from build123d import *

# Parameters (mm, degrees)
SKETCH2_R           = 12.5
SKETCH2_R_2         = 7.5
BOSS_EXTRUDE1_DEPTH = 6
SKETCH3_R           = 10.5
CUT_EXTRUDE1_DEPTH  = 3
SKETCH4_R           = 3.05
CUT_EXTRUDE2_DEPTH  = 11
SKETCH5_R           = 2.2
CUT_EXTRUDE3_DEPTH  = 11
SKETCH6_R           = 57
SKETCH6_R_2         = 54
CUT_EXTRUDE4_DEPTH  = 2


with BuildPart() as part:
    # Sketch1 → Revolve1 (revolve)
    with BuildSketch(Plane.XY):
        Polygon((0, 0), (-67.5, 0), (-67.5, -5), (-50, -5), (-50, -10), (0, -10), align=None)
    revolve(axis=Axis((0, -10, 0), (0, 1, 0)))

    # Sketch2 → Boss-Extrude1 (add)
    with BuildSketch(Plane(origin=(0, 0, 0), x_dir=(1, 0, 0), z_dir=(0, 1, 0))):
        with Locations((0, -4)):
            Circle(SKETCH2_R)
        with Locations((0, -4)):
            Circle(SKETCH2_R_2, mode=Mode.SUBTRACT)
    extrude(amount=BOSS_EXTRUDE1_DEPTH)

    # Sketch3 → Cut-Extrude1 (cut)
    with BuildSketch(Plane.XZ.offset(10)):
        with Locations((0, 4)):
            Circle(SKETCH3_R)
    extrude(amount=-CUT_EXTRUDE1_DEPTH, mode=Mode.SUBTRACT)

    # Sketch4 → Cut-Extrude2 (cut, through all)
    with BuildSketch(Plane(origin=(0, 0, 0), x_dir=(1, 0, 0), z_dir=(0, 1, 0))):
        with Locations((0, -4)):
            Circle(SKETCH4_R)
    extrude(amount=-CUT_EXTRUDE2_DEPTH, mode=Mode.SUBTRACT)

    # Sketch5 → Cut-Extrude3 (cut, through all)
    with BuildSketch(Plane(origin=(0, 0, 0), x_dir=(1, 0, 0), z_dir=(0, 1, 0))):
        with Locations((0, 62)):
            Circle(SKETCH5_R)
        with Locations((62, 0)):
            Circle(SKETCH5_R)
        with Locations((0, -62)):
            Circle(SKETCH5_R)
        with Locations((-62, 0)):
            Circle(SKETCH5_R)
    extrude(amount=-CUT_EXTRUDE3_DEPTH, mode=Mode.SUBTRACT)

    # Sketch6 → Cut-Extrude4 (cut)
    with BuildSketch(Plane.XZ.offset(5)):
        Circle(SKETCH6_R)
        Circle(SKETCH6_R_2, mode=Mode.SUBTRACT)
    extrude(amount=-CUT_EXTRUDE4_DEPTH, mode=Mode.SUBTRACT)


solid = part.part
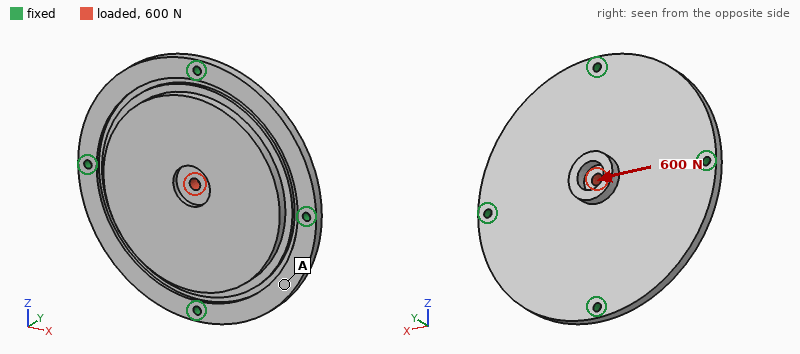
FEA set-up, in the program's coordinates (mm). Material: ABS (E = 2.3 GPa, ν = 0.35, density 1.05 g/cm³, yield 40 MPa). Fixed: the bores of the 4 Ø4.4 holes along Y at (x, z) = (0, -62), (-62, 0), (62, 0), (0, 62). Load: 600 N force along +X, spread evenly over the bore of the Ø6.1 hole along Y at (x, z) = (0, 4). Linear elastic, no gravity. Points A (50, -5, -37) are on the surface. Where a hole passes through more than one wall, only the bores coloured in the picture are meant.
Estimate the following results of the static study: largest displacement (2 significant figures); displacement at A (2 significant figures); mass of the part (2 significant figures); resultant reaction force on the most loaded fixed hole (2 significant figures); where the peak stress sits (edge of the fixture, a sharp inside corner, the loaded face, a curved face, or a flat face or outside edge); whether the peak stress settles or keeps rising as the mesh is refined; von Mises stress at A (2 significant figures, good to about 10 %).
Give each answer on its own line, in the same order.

47 µm
19 µm
110 g
170 N
edge of the fixture
keeps rising
0.40 MPa
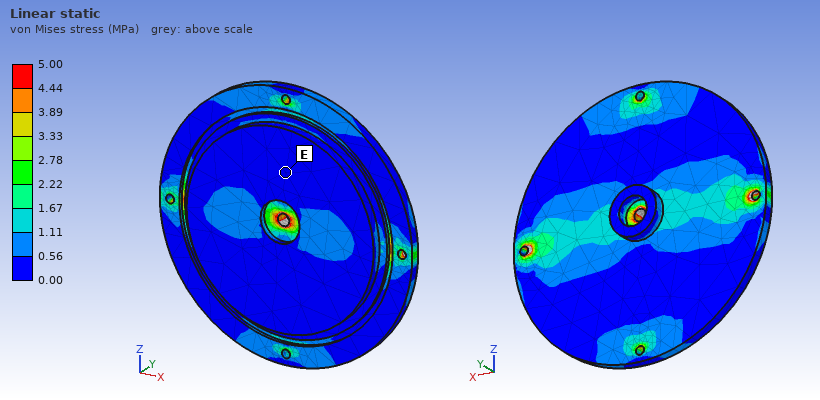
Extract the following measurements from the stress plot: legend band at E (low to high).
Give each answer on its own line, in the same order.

0.00 to 0.56 MPa
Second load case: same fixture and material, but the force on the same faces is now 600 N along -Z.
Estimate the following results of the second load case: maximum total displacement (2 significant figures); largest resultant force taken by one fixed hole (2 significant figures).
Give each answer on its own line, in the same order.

47 µm
170 N
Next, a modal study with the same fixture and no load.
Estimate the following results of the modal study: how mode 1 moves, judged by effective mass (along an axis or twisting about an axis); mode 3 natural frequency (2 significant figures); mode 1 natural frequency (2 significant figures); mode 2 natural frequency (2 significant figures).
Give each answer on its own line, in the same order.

along Y
1100 Hz
810 Hz
1100 Hz
